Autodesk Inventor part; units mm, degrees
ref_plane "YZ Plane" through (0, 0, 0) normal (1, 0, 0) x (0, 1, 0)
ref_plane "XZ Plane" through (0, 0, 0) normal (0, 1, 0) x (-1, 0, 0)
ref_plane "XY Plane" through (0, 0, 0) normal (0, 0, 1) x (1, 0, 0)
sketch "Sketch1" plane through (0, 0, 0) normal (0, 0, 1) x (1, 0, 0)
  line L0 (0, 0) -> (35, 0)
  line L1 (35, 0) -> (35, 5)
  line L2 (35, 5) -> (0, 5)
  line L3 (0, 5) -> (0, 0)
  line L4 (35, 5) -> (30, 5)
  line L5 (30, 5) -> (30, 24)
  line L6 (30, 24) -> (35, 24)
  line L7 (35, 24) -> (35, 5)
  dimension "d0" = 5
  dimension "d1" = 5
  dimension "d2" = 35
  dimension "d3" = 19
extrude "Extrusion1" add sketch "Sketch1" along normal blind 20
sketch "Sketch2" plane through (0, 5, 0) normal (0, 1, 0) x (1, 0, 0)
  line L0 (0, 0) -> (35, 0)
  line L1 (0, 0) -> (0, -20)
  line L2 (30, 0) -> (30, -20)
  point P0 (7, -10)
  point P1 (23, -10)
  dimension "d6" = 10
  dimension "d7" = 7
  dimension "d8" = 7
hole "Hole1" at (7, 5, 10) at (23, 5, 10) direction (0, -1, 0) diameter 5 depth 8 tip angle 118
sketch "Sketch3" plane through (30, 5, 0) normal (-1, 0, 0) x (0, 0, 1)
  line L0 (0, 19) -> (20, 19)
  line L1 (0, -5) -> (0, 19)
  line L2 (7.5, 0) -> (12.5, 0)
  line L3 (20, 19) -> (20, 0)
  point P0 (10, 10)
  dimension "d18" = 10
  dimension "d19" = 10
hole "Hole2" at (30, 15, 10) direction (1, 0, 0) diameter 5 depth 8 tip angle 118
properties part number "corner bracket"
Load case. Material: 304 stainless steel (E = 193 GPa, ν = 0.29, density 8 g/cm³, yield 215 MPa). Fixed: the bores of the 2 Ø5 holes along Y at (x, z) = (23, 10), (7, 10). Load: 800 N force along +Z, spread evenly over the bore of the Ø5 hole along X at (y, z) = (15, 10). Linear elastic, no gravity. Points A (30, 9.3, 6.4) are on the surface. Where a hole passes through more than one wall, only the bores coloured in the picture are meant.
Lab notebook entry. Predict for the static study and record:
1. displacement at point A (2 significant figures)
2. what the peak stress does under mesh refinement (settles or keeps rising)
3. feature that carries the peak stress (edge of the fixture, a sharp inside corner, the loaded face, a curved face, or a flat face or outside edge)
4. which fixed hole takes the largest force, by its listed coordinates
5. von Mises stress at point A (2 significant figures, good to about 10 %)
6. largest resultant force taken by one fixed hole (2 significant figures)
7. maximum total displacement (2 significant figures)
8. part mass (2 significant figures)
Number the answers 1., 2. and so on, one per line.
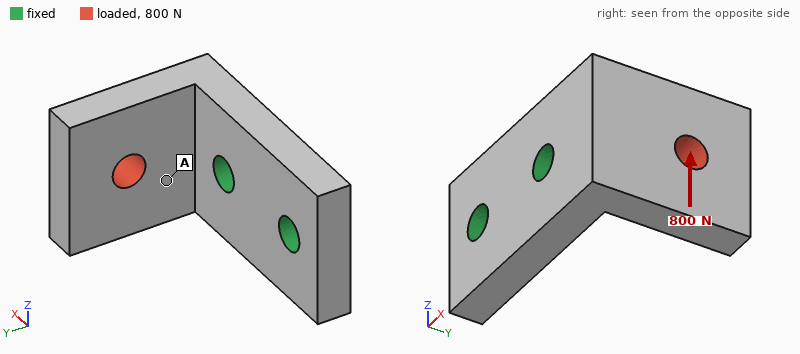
1. 11 µm
2. keeps rising
3. edge of the fixture
4. (23, 10)
5. 31 MPa
6. 1.1 kN
7. 33 µm
8. 41 g
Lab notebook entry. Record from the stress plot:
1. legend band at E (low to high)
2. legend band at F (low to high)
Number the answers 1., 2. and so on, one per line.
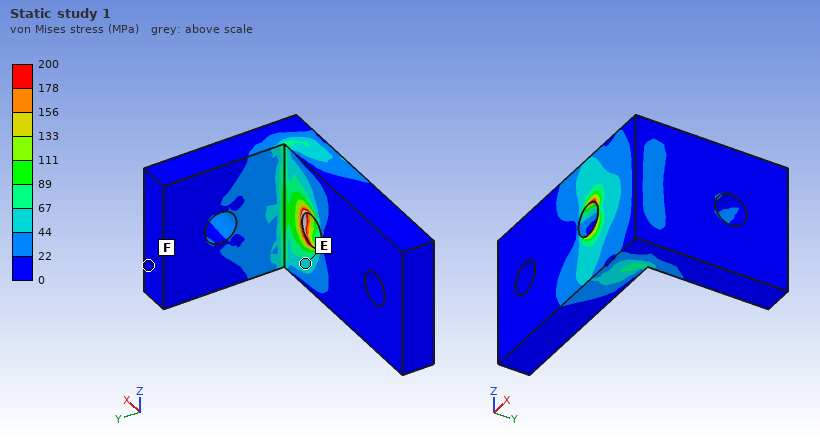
1. 44 to 67 MPa
2. 0 to 22 MPa
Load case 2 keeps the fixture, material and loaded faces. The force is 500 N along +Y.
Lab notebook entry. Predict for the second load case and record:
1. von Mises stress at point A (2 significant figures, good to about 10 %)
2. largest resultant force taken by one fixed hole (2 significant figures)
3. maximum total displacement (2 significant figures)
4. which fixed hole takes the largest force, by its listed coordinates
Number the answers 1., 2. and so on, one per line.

1. 7.3 MPa
2. 560 N
3. 13 µm
4. (23, 10)
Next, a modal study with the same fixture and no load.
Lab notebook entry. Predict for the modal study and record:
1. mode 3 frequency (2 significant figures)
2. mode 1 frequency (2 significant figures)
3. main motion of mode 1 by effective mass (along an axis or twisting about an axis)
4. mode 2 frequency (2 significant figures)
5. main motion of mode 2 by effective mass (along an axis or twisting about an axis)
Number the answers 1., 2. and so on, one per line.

1. 16 kHz
2. 5400 Hz
3. along X
4. 7600 Hz
5. along Z
